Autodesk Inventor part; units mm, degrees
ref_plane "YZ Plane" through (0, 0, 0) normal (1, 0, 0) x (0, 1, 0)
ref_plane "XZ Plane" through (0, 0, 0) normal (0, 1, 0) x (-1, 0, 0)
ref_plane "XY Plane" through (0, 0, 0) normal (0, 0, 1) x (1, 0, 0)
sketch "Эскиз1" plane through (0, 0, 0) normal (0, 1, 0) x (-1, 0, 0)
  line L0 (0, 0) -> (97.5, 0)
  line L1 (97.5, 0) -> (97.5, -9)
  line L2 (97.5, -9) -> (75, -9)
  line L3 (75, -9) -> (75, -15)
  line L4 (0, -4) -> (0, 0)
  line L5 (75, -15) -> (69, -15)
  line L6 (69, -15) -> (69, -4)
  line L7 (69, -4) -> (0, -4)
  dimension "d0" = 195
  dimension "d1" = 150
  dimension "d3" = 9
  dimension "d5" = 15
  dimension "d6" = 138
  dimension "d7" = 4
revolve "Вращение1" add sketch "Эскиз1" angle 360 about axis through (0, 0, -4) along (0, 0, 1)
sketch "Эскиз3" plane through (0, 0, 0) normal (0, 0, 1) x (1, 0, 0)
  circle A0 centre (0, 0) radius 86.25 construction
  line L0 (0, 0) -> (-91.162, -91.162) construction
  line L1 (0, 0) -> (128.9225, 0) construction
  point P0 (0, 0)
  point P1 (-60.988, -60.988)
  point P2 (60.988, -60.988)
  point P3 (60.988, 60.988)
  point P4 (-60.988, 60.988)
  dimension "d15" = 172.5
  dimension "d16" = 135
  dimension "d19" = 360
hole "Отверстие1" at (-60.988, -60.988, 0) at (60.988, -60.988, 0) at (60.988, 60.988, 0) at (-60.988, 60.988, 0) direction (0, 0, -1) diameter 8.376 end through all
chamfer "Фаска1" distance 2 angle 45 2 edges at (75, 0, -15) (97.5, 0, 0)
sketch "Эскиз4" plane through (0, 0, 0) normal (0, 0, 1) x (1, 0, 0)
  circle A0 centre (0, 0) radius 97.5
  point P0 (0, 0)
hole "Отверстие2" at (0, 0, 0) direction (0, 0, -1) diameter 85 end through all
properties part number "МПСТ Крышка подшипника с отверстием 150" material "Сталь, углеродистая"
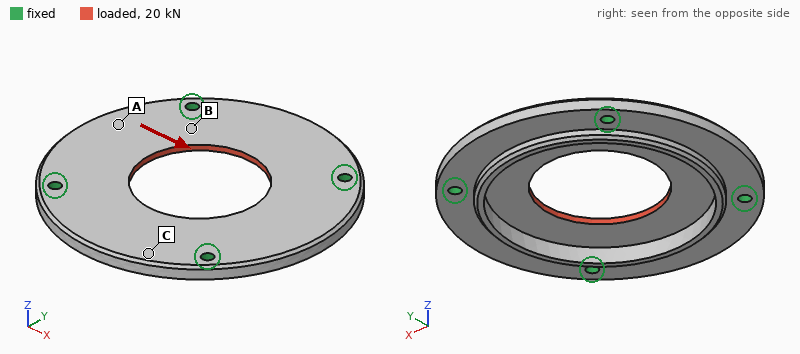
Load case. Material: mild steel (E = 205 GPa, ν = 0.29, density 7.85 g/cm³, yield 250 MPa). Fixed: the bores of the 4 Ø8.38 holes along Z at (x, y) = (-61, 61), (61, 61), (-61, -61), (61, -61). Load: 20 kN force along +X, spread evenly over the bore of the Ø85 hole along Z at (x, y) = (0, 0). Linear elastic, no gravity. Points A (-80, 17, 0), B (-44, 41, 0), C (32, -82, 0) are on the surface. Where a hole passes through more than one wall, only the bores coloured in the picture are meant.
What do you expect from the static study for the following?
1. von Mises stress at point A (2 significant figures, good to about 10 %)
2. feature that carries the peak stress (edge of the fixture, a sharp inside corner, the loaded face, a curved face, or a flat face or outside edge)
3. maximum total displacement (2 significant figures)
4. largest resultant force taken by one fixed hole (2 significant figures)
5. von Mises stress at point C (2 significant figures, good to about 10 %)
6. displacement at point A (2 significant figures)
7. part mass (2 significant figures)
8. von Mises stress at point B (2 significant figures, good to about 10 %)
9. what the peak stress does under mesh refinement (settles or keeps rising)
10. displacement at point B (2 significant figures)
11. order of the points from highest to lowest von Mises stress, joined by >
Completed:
13 MPa
edge of the fixture
15 µm
5.0 kN
3.8 MPa
7.8 µm
1.4 kg
22 MPa
keeps rising
5.8 µm
B > A > C
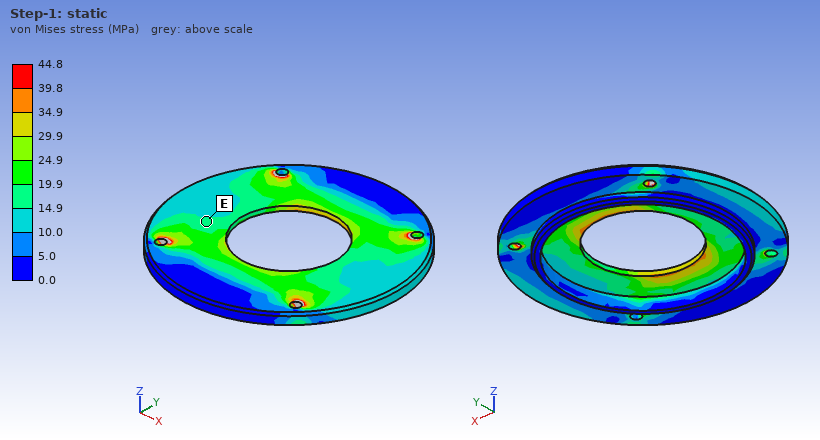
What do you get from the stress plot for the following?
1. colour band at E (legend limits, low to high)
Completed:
14.9 to 19.9 MPa
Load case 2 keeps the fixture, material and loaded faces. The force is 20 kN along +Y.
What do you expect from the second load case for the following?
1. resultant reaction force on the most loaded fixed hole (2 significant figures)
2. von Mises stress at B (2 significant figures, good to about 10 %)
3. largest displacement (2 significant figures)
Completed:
5.0 kN
23 MPa
15 µm
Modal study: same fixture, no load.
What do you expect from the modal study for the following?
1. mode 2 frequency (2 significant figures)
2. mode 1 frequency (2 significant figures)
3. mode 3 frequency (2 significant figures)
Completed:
2900 Hz
2600 Hz
2900 Hz
